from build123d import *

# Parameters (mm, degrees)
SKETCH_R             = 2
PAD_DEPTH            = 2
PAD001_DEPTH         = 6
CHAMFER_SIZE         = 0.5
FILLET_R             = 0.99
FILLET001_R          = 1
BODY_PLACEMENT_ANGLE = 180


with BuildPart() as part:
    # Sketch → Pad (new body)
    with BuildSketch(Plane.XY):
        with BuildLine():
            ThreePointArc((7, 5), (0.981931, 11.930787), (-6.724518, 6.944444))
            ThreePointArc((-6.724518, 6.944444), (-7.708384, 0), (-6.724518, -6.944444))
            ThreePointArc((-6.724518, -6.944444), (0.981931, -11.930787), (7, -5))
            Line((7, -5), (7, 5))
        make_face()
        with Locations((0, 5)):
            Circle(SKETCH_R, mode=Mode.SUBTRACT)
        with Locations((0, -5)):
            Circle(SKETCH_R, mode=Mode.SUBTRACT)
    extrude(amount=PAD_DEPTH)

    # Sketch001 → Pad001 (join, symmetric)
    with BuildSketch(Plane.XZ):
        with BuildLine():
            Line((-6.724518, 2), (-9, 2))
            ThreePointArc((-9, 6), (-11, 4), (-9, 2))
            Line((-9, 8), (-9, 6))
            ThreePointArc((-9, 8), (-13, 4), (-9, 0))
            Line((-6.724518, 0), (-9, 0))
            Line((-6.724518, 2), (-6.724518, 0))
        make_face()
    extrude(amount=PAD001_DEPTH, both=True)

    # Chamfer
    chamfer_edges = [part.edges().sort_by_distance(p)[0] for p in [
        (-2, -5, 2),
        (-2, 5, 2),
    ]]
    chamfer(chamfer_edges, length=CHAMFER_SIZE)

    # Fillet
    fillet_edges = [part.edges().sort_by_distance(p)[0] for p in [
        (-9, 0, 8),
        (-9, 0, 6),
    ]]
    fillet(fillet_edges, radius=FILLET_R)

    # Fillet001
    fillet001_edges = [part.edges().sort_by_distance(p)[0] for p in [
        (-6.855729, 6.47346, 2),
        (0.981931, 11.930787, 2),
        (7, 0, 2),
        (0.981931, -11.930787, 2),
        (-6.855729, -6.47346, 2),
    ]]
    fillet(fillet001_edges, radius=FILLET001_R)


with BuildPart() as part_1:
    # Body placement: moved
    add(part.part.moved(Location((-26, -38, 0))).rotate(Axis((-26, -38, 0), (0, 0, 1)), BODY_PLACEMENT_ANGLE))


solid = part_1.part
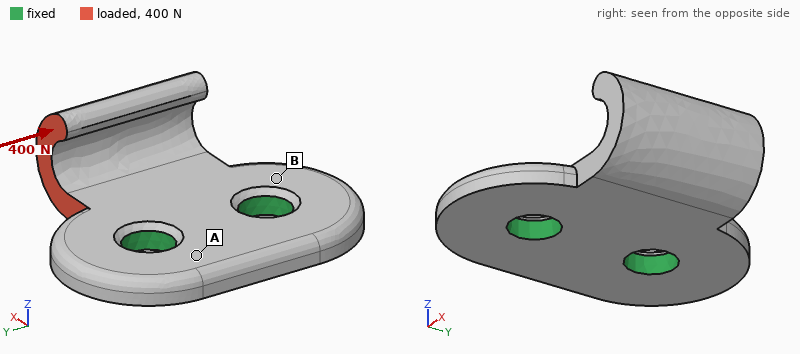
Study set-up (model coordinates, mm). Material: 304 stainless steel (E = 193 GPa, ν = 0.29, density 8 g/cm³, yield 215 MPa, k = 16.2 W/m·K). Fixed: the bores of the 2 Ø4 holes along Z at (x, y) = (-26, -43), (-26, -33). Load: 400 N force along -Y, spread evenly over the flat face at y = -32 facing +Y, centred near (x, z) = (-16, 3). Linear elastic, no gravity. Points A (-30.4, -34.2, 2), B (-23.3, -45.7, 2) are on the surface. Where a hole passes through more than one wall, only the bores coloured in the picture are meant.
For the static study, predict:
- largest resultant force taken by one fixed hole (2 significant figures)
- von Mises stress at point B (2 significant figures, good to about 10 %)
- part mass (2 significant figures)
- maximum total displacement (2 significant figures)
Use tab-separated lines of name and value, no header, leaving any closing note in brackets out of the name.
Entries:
largest resultant force taken by one fixed hole	380 N
von Mises stress at point B	24 MPa
part mass	6.3 g
maximum total displacement	22 µm
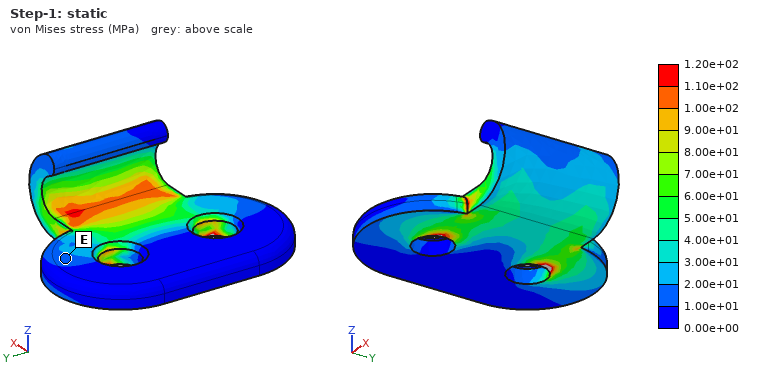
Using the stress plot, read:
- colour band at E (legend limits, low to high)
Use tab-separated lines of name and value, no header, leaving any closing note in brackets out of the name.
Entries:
colour band at E	1.00e+01 to 2.00e+01 MPa
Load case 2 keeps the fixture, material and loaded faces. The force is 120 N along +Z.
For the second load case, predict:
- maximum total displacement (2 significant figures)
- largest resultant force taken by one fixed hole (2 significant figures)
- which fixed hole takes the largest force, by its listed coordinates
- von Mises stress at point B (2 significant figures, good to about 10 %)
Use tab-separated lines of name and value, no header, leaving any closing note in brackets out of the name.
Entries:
maximum total displacement	35 µm
largest resultant force taken by one fixed hole	120 N
which fixed hole takes the largest force, by its listed coordinates	(-26, -33)
von Mises stress at point B	25 MPa
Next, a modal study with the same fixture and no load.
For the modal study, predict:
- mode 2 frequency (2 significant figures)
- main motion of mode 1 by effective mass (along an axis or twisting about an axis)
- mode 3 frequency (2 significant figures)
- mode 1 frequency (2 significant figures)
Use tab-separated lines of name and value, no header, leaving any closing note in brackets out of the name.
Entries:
mode 2 frequency	15 kHz
main motion of mode 1 by effective mass	along Z
mode 3 frequency	23 kHz
mode 1 frequency	7700 Hz
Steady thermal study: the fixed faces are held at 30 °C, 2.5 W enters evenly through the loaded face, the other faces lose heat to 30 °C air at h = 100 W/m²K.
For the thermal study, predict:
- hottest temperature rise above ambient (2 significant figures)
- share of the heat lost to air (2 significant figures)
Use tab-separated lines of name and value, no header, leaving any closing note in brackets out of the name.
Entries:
hottest temperature rise above ambient	61 K
share of the heat lost to air	46 %
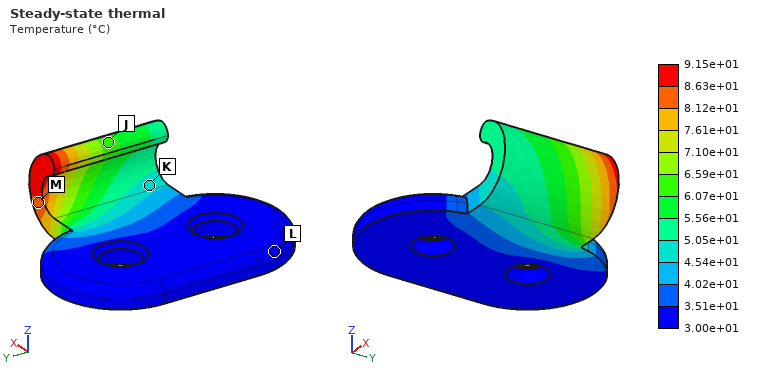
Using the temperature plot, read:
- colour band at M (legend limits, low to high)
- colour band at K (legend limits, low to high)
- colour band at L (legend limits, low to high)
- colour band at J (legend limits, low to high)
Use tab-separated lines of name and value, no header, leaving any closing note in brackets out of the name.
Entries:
colour band at M	8.12e+01 to 8.63e+01 °C
colour band at K	4.54e+01 to 5.05e+01 °C
colour band at L	3.00e+01 to 3.51e+01 °C
colour band at J	6.07e+01 to 6.59e+01 °C
